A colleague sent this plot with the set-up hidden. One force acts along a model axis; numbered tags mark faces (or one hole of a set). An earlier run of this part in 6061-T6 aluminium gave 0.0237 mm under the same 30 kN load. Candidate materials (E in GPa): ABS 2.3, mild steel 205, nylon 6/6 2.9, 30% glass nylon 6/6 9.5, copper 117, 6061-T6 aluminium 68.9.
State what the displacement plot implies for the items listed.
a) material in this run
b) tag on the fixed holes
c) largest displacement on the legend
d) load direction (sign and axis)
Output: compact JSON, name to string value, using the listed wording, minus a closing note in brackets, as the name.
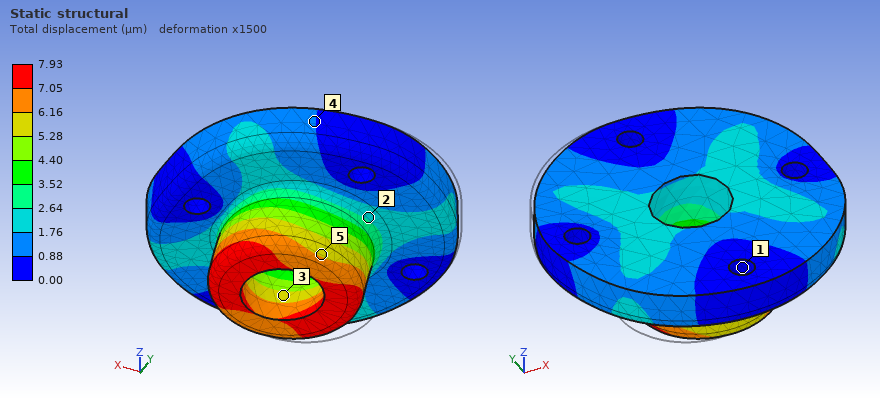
{"material in this run": "mild steel", "tag on the fixed holes": "1", "largest displacement on the legend": "7.93 µm", "load direction": "+X"}
